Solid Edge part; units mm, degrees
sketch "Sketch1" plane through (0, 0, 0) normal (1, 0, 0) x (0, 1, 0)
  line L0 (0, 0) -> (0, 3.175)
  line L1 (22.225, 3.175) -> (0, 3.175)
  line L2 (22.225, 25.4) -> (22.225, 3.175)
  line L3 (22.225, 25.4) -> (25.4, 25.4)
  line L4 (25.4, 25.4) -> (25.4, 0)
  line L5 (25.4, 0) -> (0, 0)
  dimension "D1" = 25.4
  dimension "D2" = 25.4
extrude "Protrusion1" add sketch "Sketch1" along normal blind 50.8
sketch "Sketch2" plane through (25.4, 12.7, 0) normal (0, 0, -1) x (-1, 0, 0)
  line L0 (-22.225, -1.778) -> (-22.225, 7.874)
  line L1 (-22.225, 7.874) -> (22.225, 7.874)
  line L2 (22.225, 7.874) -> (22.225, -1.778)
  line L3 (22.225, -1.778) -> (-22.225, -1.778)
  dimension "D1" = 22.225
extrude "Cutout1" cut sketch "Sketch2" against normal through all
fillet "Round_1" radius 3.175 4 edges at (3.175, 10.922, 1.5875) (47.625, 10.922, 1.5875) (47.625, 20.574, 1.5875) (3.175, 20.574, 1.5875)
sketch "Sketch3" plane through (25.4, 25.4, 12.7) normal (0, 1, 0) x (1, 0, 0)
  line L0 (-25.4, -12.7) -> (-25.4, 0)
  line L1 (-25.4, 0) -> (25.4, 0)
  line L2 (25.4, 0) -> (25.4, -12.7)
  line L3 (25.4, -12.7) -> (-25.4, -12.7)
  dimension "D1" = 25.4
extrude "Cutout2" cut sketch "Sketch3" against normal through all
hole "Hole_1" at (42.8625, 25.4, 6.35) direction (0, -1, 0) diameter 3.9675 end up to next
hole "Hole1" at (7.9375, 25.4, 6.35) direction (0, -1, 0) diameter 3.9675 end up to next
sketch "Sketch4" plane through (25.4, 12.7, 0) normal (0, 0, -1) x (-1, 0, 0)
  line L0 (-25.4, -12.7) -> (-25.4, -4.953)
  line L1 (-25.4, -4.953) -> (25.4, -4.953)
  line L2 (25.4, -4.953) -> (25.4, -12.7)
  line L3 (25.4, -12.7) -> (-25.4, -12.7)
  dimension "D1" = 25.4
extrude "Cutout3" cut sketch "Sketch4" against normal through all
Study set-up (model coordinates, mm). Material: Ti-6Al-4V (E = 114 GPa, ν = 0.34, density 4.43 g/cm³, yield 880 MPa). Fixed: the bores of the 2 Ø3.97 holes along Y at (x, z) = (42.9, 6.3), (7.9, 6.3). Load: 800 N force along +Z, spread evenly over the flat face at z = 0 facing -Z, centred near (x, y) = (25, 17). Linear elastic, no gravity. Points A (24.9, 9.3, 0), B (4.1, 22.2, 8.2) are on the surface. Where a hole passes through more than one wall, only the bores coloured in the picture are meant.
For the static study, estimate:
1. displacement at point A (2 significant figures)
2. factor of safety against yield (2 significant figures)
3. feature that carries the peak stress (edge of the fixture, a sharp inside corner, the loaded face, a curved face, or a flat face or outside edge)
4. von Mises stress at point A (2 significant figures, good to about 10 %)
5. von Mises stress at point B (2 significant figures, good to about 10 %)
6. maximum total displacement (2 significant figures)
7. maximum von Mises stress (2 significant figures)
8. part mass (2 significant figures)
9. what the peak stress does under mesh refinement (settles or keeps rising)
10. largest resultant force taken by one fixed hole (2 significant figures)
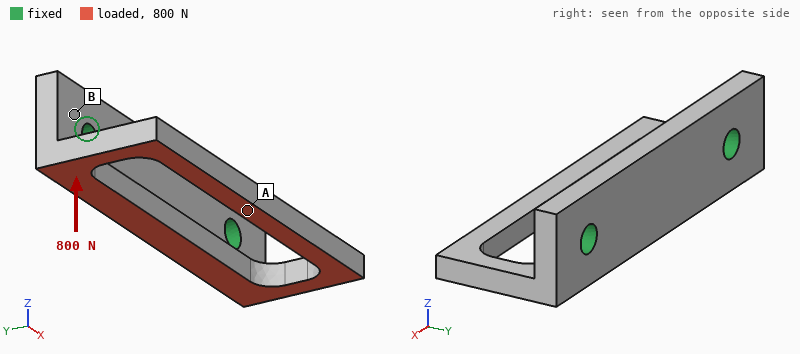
0.34 mm
2.8
the loaded face
160 MPa
34 MPa
0.37 mm
310 MPa
13 g
settles
400 N
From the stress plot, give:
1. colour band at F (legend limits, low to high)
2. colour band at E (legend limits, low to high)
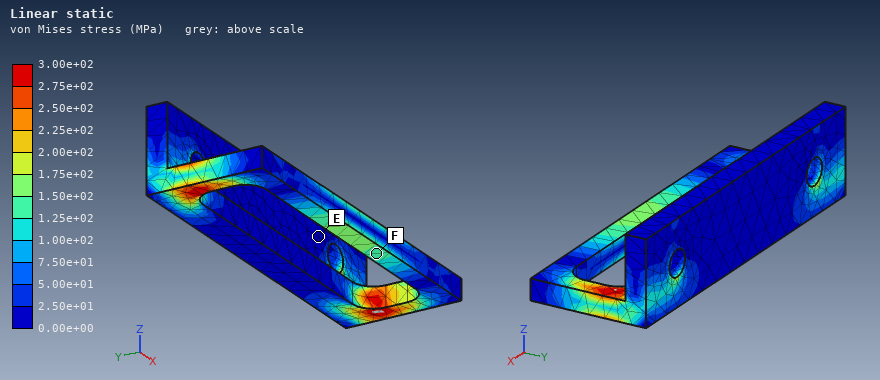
1.25e+02 to 1.50e+02 MPa
0.00e+00 to 2.50e+01 MPa
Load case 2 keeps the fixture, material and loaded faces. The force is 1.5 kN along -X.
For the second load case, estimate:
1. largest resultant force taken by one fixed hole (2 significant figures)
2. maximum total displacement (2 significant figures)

790 N
0.13 mm
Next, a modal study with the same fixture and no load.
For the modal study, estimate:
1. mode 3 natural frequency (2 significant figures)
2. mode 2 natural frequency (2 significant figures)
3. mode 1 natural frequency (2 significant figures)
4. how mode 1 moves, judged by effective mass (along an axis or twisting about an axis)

6800 Hz
6500 Hz
3400 Hz
along Z
